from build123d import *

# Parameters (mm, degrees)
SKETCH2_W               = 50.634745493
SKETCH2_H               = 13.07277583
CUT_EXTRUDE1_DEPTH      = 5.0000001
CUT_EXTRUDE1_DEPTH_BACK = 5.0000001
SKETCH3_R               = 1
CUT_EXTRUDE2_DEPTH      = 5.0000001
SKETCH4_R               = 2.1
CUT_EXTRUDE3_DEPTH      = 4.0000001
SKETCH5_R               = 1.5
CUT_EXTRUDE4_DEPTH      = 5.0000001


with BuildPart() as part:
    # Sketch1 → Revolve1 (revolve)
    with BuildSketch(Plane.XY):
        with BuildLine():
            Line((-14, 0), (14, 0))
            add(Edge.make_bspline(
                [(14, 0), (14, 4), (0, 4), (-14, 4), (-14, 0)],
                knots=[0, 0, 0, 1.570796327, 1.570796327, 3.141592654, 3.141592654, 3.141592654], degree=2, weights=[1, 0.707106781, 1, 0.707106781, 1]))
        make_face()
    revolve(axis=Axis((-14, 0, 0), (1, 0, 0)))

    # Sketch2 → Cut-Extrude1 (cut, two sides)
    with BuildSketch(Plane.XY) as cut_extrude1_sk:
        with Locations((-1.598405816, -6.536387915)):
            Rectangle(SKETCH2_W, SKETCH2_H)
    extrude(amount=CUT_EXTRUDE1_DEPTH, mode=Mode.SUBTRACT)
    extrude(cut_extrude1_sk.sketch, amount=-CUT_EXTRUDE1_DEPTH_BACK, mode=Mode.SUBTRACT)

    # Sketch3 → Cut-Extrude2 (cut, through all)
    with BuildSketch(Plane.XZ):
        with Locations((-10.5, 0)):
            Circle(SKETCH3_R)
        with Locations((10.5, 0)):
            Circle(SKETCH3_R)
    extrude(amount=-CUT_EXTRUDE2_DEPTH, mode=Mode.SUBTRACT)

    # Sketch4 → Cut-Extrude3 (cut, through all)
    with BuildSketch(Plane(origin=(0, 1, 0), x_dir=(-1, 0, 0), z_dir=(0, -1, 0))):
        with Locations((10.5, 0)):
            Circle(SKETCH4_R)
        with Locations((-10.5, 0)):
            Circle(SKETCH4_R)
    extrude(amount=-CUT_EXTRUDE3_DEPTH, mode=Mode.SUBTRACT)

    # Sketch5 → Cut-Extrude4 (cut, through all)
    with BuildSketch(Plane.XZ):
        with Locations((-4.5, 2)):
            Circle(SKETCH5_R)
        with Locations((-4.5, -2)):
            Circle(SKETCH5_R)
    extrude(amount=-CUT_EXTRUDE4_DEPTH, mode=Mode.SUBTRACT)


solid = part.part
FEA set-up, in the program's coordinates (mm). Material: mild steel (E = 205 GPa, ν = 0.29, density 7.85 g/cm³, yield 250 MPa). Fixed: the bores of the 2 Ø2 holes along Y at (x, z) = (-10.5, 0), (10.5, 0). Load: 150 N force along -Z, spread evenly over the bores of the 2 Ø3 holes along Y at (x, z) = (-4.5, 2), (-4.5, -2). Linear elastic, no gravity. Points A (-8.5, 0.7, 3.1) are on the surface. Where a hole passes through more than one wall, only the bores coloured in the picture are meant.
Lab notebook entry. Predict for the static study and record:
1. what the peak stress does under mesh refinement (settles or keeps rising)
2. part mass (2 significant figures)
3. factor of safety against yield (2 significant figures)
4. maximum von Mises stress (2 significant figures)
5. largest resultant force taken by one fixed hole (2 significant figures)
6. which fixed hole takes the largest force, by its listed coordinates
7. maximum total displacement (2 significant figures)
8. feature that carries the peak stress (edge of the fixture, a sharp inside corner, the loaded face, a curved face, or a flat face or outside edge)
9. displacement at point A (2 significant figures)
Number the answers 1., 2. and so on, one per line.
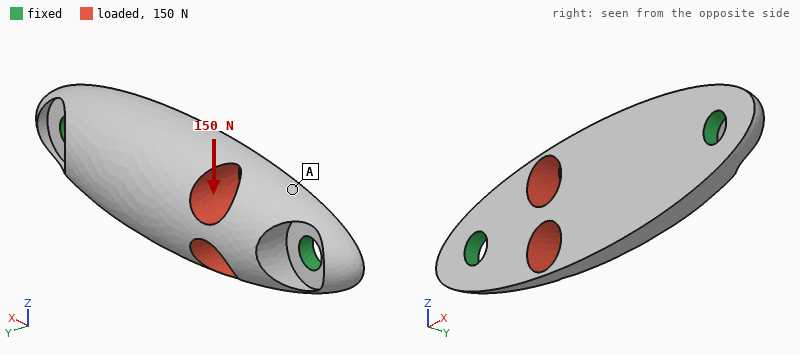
1. settles
2. 3.0 g
3. 0.69
4. 360 MPa
5. 110 N
6. (-10.5, 0)
7. 4.0 µm
8. the loaded face
9. 1.8 µm
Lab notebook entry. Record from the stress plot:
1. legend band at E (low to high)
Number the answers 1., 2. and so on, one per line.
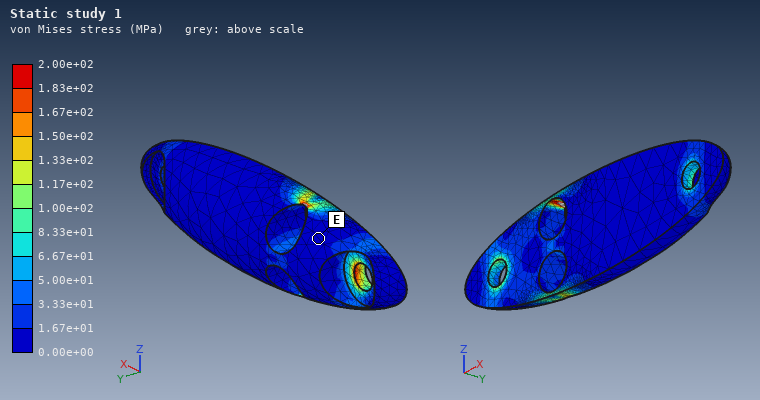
1. 0.00e+00 to 1.67e+01 MPa
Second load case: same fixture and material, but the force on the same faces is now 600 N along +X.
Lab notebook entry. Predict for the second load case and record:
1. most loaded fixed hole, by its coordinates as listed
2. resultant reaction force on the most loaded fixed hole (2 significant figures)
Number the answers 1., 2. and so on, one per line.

1. (-10.5, 0)
2. 320 N
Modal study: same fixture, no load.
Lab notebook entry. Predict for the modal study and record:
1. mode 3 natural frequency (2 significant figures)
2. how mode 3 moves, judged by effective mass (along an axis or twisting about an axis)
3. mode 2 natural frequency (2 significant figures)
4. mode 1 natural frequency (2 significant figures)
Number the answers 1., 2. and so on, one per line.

1. 30 kHz
2. along Z
3. 23 kHz
4. 22 kHz
